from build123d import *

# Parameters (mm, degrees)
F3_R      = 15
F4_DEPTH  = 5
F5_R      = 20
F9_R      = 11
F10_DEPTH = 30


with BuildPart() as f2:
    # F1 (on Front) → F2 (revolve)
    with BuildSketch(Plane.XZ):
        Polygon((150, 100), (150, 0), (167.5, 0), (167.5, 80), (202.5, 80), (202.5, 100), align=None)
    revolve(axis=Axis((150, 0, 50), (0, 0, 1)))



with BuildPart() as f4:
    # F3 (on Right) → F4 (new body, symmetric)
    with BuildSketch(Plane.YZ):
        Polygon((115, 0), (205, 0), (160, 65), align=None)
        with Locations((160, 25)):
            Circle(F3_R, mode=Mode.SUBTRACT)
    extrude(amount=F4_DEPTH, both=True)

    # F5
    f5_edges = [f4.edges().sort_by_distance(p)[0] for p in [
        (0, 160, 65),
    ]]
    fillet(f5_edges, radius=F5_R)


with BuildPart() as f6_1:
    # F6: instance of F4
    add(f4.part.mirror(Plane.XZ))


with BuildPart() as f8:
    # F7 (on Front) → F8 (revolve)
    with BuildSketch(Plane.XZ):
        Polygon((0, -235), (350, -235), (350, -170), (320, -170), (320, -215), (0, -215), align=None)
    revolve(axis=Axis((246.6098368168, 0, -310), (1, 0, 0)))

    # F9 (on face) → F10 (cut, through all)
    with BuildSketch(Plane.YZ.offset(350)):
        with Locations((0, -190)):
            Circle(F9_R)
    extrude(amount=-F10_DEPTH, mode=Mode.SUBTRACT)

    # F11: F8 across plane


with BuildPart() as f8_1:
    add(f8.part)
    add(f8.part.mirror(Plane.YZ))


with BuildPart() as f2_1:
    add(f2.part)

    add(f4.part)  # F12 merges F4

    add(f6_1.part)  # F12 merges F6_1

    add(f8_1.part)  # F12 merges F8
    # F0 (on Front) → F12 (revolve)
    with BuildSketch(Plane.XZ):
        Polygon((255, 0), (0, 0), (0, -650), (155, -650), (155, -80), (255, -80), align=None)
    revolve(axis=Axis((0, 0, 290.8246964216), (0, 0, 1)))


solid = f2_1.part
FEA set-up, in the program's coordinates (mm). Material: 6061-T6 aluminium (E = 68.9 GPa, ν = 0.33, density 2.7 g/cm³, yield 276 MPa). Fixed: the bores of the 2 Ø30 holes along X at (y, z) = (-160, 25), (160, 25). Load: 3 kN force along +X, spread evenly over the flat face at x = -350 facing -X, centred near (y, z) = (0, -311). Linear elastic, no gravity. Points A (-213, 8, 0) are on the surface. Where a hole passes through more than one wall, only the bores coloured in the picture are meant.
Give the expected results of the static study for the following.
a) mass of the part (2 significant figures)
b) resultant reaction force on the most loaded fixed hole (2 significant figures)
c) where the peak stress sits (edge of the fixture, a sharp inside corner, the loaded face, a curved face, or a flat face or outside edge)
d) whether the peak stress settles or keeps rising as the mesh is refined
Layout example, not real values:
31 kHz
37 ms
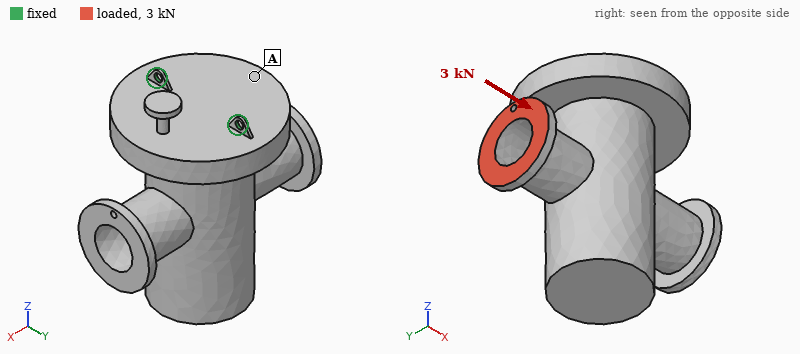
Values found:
180 kg
1.5 kN
edge of the fixture
keeps rising
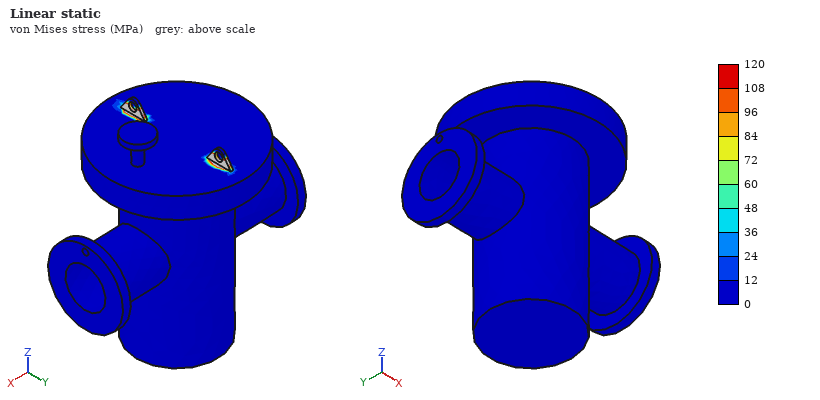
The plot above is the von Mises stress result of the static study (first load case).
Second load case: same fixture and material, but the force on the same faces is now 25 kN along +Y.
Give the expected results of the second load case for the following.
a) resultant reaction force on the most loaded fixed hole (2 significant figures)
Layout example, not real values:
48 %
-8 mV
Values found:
39 kN
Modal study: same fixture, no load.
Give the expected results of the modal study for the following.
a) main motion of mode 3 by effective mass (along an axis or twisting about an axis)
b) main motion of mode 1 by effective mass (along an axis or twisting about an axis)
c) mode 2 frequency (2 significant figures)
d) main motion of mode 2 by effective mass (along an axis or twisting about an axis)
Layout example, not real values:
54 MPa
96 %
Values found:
twisting about Z
along X
230 Hz
along Y
